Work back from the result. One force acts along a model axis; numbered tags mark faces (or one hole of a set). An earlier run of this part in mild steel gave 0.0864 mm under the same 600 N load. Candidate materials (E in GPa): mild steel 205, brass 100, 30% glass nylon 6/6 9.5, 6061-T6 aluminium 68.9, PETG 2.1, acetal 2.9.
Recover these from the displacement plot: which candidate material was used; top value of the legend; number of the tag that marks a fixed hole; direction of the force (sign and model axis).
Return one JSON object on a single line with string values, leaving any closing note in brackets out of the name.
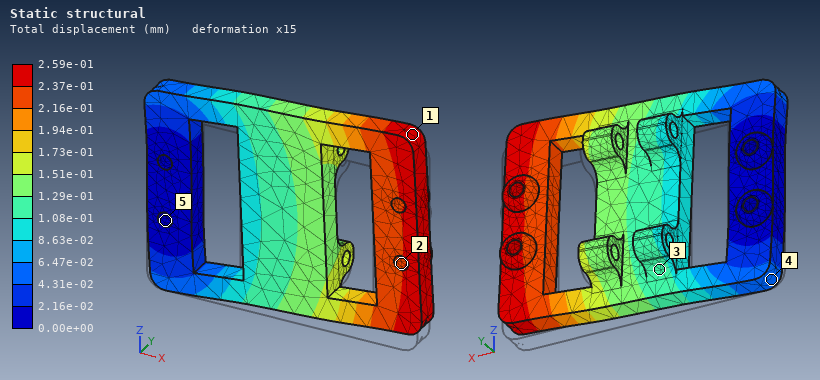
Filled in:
{"which candidate material was used": "6061-T6 aluminium", "top value of the legend": "2.59e-01 mm", "number of the tag that marks a fixed hole": "5", "direction of the force": "+Z"}
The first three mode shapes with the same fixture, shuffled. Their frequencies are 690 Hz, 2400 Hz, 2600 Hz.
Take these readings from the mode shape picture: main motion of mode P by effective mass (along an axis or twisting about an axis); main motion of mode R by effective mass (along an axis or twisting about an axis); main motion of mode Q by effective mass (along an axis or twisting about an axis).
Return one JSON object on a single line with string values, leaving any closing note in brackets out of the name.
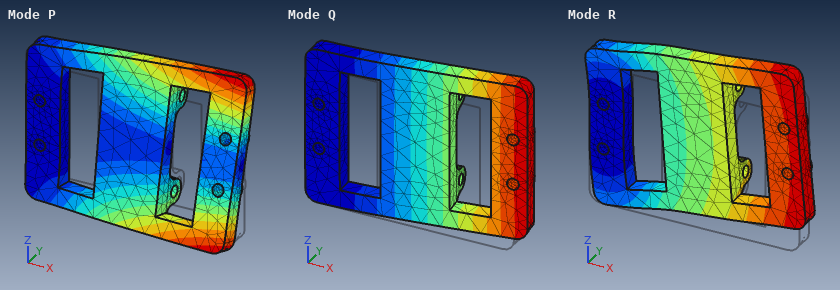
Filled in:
{"main motion of mode P by effective mass": "twisting about X", "main motion of mode R by effective mass": "along Z", "main motion of mode Q by effective mass": "along Y"}
